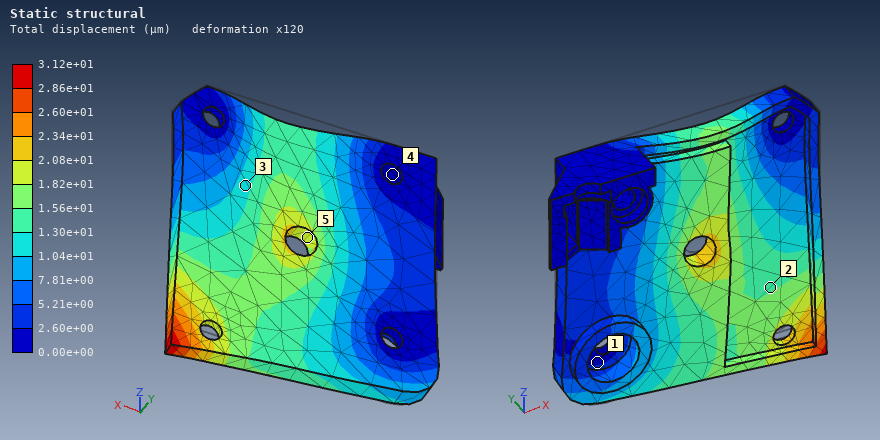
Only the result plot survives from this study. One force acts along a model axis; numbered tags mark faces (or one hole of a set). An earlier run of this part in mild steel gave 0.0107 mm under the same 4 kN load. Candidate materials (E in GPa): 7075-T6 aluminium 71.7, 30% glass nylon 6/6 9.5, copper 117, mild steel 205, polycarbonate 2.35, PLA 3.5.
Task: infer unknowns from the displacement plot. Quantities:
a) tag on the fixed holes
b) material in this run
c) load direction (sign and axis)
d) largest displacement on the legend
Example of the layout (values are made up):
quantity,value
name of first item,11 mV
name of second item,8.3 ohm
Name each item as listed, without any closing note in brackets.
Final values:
quantity,value
tag on the fixed holes,4
material in this run,7075-T6 aluminium
load direction,-Z
largest displacement on the legend,3.12e+01 µm
